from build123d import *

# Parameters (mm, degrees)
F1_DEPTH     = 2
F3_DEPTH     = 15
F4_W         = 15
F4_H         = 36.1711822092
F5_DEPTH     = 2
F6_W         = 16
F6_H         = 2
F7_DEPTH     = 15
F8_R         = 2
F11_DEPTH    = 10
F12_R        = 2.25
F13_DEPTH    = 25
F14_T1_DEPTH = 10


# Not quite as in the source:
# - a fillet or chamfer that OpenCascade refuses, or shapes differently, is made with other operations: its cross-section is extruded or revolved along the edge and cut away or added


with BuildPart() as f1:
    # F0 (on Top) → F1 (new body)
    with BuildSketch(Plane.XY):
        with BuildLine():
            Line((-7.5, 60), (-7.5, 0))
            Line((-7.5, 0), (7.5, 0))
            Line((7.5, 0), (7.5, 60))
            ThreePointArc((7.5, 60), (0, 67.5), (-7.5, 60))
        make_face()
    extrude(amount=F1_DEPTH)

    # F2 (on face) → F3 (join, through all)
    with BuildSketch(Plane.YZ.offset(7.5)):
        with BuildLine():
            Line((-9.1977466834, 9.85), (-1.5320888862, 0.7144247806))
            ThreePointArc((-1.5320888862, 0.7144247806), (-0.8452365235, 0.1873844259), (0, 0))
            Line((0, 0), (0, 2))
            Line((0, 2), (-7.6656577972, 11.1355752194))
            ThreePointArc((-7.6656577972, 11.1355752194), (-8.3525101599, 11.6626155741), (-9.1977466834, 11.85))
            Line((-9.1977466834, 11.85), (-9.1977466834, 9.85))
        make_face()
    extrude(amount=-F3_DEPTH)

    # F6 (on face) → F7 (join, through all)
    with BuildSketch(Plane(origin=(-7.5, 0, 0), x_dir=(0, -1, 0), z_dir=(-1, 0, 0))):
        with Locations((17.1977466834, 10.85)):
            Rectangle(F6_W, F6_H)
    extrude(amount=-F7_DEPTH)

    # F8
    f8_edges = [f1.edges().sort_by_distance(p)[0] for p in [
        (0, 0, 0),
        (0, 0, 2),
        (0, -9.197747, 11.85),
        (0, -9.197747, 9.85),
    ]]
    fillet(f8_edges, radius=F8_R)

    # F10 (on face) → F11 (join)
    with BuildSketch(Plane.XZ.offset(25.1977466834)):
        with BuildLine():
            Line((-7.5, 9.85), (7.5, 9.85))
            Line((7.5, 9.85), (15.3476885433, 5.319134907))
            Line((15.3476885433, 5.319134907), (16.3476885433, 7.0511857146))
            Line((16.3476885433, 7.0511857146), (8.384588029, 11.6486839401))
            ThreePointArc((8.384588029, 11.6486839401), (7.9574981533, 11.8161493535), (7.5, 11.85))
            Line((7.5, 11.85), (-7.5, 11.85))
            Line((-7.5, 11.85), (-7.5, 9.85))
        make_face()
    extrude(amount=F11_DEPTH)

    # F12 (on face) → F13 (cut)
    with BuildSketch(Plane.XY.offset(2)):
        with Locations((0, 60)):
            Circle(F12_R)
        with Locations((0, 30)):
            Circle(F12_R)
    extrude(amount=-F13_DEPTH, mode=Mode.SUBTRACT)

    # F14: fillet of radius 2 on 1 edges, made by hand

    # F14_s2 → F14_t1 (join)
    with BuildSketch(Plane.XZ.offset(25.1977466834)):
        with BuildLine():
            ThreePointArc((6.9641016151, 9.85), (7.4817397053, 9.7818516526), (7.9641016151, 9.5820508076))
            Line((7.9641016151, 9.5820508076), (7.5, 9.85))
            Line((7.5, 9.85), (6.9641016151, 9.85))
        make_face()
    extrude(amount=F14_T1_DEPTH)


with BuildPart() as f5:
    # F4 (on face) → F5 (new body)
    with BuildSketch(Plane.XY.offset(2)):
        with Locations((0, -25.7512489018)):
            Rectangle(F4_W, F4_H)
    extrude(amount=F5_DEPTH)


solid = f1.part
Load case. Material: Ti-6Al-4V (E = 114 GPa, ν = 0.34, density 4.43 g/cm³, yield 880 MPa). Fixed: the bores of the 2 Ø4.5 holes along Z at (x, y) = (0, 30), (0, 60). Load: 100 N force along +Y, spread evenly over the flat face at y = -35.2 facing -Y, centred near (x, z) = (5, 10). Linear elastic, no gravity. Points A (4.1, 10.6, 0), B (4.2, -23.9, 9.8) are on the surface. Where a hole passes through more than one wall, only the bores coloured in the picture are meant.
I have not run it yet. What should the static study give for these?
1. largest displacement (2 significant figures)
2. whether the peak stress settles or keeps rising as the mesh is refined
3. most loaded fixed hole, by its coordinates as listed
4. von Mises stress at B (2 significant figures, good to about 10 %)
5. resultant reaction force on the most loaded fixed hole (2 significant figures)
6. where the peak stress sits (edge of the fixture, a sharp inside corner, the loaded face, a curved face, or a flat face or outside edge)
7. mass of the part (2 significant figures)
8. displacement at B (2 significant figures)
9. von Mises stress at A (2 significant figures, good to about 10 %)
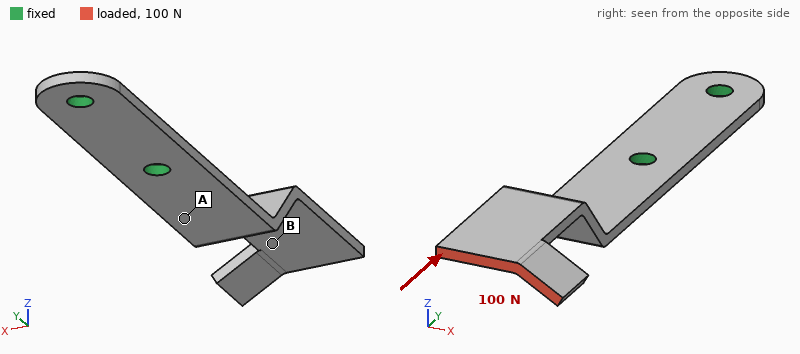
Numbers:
1.3 mm
keeps rising
(0, 30)
16 MPa
94 N
edge of the fixture
15 g
0.96 mm
82 MPa
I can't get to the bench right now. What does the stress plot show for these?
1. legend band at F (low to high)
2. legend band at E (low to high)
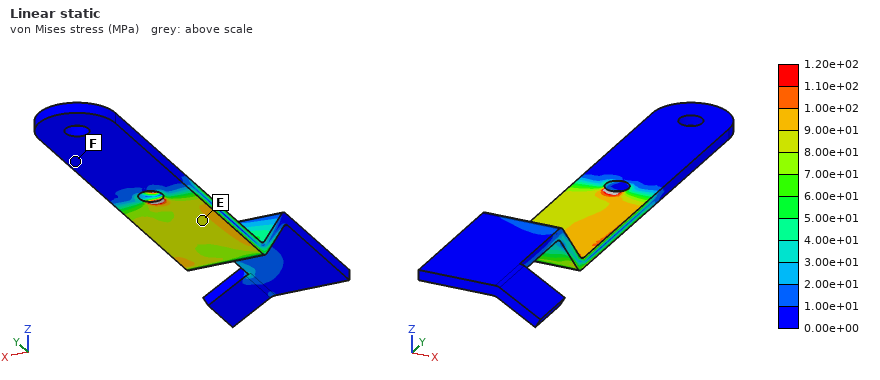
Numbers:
0.00e+00 to 1.00e+01 MPa
8.00e+01 to 9.00e+01 MPa
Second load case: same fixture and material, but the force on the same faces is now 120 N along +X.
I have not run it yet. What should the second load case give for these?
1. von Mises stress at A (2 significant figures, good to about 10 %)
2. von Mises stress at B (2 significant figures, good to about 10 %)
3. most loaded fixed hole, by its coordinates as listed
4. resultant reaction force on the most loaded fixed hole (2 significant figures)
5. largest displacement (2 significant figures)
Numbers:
90 MPa
24 MPa
(0, 30)
260 N
0.67 mm
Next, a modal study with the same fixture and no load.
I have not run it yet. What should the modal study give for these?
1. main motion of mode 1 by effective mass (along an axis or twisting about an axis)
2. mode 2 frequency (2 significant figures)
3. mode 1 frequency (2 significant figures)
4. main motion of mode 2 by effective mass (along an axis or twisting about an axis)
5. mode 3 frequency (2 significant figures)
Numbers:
along Z
1200 Hz
340 Hz
along X
1900 Hz
